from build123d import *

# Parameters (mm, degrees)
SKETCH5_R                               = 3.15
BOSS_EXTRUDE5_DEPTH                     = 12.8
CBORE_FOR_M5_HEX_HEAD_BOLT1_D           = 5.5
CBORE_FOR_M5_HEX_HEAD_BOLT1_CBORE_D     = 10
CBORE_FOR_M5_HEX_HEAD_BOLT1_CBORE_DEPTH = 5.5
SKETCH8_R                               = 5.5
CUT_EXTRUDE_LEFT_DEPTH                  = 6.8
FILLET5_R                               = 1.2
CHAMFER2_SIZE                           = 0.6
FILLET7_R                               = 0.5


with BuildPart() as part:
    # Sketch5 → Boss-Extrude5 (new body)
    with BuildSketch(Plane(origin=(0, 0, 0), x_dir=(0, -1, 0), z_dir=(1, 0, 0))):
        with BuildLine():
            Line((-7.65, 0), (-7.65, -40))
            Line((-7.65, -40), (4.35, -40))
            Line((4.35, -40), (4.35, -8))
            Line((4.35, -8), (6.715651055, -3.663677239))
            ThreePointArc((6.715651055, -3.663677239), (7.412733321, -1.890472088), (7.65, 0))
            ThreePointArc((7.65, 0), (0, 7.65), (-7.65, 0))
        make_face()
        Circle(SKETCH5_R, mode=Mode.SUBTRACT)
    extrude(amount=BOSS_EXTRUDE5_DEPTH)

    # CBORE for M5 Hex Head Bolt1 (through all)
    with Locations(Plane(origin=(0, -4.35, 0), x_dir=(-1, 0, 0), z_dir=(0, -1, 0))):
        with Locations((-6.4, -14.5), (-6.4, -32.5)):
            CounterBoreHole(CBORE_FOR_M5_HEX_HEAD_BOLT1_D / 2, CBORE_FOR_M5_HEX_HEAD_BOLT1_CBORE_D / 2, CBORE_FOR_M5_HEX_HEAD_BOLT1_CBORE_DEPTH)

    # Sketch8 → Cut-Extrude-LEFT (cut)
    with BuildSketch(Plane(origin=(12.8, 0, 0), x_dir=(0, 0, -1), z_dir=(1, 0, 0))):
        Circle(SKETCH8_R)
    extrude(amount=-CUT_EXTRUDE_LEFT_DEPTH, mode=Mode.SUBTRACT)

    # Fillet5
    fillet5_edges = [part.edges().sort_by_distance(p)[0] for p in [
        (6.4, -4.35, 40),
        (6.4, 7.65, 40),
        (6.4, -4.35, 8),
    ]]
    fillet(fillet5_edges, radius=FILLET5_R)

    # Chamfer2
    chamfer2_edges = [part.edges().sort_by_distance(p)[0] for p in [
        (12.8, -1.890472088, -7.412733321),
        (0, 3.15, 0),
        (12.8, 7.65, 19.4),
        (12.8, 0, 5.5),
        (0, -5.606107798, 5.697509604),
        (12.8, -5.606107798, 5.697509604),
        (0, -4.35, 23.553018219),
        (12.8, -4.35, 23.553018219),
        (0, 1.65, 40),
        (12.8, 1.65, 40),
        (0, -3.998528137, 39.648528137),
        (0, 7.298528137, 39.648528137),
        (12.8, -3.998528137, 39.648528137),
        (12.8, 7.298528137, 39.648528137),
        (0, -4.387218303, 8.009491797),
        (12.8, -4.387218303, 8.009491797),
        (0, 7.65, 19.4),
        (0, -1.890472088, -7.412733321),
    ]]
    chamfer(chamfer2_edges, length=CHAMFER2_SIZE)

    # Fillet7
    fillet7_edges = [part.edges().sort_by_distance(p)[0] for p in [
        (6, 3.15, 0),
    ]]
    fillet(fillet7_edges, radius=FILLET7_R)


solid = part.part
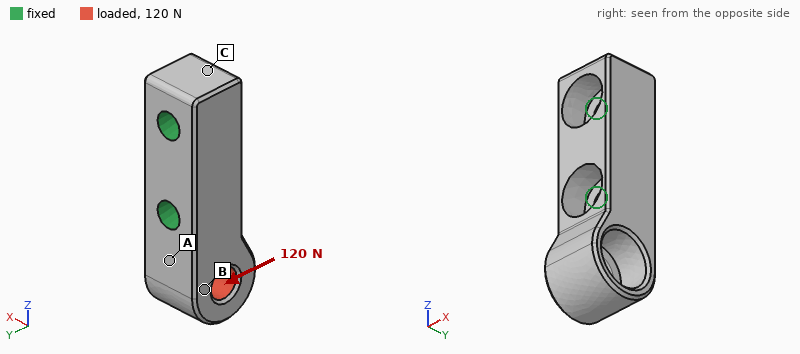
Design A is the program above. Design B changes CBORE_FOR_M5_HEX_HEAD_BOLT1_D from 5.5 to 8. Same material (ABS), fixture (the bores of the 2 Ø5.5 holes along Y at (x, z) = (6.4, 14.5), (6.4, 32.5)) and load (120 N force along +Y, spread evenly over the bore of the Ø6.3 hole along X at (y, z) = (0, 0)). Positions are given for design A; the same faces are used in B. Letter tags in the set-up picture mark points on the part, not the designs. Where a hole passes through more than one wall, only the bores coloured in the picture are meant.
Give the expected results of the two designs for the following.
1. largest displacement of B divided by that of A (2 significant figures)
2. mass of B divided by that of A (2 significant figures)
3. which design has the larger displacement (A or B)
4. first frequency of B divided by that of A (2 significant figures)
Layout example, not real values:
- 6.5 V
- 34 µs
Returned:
- 0.78
- 0.94
- A
- 1.1
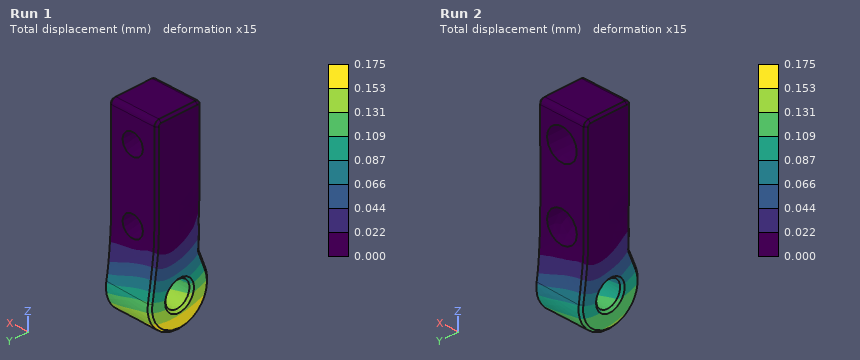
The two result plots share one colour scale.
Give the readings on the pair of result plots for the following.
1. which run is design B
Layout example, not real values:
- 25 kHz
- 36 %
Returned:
- Run 2
